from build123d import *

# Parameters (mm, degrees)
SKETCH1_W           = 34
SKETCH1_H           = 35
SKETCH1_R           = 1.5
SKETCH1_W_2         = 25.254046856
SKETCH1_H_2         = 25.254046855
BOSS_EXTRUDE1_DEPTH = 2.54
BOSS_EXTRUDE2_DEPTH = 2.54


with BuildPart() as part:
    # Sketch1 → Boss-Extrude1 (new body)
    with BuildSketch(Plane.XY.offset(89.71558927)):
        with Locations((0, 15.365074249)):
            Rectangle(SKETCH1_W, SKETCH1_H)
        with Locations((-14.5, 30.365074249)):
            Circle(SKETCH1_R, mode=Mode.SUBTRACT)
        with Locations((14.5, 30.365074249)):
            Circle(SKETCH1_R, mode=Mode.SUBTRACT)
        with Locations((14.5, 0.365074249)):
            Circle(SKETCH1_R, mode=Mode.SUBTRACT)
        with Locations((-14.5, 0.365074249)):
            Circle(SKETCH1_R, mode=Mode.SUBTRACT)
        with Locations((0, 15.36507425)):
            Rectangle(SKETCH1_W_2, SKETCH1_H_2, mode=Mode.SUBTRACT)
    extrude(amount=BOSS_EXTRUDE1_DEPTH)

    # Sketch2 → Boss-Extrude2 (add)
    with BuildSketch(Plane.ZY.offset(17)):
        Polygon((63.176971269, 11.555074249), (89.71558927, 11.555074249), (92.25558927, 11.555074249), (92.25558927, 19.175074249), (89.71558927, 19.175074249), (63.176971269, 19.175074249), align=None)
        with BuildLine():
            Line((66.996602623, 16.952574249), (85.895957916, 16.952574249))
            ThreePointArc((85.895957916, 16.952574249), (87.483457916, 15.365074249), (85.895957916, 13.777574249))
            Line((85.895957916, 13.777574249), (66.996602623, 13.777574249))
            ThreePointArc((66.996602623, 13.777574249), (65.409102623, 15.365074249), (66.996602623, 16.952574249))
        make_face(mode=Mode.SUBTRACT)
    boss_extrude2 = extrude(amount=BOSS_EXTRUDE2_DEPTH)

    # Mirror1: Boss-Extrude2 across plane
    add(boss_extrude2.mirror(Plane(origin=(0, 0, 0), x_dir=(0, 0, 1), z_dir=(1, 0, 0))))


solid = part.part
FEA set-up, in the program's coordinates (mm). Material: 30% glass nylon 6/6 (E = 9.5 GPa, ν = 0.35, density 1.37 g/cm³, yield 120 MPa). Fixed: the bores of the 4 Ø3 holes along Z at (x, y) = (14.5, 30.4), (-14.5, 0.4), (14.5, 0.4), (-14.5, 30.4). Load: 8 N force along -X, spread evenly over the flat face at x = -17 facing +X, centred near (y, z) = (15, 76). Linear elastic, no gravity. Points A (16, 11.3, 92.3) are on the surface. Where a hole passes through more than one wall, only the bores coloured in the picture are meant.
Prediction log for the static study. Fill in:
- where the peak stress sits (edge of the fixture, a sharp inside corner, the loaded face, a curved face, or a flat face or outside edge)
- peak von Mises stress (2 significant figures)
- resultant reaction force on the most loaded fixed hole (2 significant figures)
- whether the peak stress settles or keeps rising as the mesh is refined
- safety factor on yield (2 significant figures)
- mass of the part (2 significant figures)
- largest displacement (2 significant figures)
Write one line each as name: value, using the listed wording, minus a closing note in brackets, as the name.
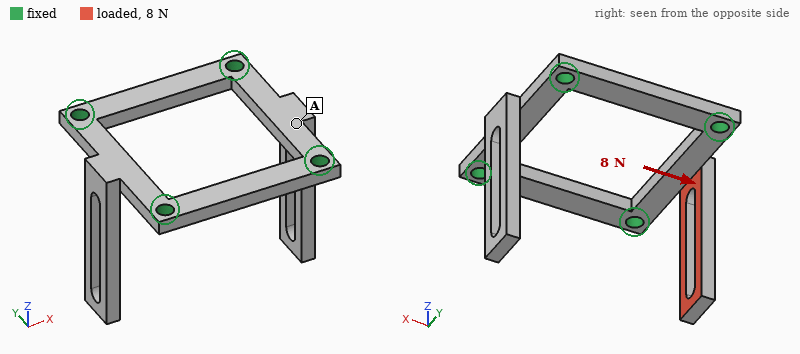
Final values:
where the peak stress sits: the loaded face
peak von Mises stress: 22 MPa
resultant reaction force on the most loaded fixed hole: 4.3 N
whether the peak stress settles or keeps rising as the mesh is refined: settles
safety factor on yield: 5.4
mass of the part: 2.9 g
largest displacement: 0.72 mm
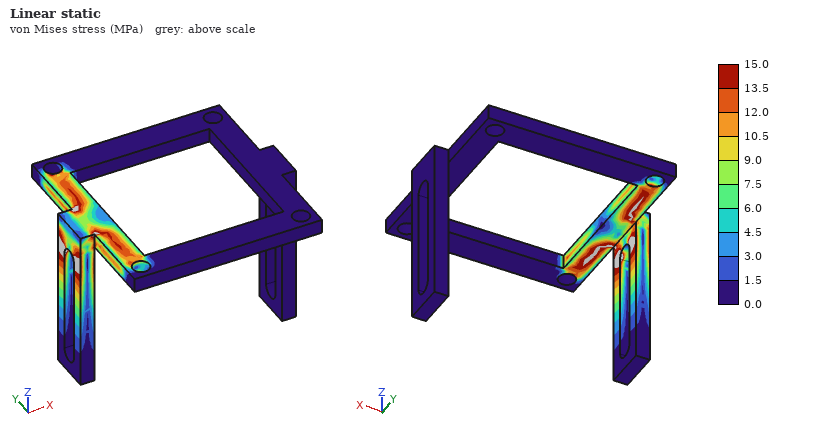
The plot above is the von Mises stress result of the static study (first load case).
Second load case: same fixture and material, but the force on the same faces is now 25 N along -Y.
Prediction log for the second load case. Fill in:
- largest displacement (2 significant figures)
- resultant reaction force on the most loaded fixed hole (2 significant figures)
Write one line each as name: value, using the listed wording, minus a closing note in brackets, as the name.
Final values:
largest displacement: 0.62 mm
resultant reaction force on the most loaded fixed hole: 23 N
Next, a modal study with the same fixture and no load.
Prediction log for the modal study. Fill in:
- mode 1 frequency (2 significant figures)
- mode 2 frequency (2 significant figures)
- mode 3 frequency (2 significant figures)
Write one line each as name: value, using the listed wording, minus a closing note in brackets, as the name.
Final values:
mode 1 frequency: 940 Hz
mode 2 frequency: 940 Hz
mode 3 frequency: 1700 Hz
